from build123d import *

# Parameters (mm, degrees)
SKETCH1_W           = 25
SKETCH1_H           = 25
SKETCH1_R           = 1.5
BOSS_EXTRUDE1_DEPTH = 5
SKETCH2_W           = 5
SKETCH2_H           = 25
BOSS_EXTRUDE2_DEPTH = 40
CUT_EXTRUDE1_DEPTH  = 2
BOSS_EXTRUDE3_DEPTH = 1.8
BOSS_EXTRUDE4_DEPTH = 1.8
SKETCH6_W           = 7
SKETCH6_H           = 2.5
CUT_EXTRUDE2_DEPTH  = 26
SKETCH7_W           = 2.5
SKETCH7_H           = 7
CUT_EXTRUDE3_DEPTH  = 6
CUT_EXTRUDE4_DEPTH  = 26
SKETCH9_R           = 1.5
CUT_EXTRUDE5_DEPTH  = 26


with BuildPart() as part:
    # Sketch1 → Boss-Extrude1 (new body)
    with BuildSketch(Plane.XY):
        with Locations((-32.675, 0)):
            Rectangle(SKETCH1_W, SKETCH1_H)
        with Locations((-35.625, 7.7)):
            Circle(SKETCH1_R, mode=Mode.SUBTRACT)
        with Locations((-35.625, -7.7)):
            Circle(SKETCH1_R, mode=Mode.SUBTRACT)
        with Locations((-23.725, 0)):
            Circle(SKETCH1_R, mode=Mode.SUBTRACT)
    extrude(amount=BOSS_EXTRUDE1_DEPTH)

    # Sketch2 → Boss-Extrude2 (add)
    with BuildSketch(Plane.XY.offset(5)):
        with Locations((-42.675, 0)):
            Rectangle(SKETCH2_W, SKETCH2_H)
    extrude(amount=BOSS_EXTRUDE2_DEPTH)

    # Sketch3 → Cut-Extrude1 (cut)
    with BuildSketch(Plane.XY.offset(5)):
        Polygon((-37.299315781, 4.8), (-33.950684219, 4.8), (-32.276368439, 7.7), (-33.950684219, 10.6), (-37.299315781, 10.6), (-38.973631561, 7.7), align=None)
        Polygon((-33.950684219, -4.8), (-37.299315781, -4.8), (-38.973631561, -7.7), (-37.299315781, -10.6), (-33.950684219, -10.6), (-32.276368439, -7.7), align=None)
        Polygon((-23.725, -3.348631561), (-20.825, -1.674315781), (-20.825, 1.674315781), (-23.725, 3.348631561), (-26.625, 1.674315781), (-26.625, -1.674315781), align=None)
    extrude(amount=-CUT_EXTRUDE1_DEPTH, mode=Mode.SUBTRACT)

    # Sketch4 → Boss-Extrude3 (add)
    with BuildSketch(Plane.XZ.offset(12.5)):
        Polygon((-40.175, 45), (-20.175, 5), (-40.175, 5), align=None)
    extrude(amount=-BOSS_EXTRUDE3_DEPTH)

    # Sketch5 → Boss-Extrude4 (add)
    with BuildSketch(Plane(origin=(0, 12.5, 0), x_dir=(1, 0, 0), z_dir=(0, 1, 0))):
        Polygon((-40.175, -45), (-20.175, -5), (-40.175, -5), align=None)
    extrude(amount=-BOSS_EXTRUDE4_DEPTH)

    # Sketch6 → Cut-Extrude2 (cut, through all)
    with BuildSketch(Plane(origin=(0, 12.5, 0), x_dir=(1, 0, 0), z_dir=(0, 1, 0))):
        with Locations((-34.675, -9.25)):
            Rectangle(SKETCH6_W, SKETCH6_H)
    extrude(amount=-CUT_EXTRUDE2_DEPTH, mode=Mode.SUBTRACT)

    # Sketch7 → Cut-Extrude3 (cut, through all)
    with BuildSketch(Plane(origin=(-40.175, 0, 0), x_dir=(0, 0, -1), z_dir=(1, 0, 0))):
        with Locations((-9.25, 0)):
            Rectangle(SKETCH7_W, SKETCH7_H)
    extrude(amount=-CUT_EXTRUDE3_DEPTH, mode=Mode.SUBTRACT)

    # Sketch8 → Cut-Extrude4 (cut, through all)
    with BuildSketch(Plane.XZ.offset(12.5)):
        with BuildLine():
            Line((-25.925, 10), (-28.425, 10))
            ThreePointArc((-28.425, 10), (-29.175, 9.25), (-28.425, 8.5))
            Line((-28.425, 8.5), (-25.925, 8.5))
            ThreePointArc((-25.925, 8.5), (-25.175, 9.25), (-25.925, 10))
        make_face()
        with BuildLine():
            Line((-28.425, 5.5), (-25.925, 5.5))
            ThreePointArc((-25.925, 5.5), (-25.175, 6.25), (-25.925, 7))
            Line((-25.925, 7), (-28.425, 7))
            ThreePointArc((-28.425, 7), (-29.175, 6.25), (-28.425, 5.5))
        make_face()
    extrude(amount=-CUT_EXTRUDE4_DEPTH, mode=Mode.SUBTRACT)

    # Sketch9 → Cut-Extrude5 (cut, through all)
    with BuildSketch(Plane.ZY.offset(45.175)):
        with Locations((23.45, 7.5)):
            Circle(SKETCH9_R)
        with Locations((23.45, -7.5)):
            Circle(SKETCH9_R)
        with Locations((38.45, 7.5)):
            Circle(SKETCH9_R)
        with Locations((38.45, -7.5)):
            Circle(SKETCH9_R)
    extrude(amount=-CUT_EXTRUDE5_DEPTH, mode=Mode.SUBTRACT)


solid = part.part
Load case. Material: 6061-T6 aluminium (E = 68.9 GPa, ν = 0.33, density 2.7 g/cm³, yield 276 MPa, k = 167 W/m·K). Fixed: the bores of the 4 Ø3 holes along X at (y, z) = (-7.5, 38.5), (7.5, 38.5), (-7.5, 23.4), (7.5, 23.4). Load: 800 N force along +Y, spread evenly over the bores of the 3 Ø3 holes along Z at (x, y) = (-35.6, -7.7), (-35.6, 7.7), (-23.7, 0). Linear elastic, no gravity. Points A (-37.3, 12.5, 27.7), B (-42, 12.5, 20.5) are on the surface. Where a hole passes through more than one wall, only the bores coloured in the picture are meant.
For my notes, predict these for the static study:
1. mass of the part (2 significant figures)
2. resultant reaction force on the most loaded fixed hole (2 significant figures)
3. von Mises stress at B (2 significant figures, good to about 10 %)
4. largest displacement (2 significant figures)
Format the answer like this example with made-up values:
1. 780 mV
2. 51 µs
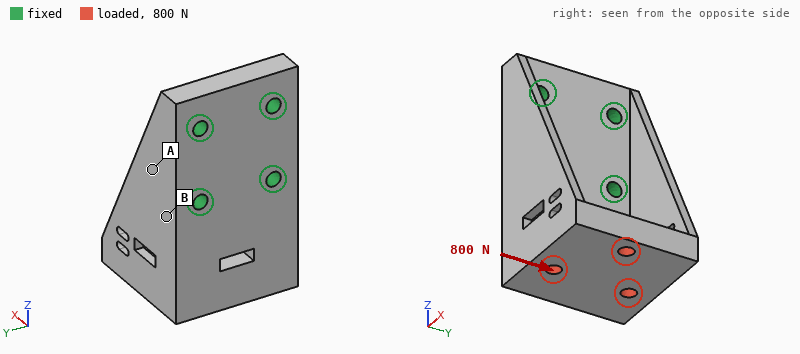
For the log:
1. 24 g
2. 1.2 kN
3. 36 MPa
4. 89 µm
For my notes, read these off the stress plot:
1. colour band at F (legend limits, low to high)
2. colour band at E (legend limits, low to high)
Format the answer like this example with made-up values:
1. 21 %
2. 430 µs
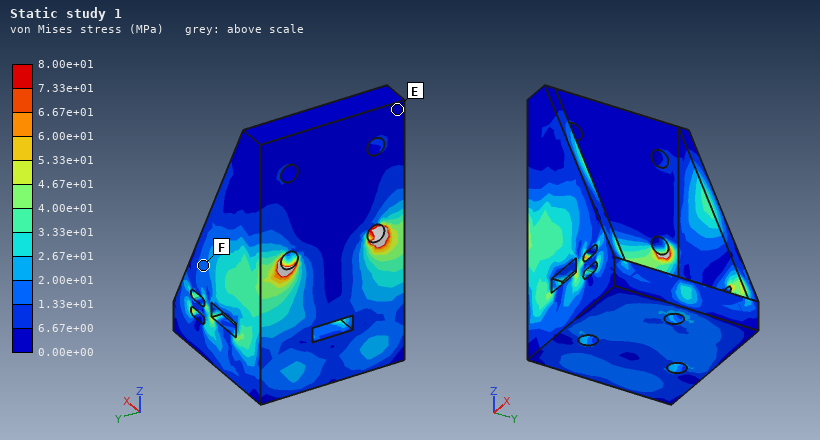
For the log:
1. 1.33e+01 to 2.00e+01 MPa
2. 0.00e+00 to 6.67e+00 MPa
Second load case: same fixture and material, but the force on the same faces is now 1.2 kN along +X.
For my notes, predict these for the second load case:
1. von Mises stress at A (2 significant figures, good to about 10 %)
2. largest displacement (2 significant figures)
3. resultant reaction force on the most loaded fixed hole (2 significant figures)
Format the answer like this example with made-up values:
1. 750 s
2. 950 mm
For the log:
1. 43 MPa
2. 0.11 mm
3. 1.2 kN
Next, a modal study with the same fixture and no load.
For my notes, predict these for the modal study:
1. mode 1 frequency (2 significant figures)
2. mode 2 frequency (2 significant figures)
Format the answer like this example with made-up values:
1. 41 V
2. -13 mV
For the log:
1. 5700 Hz
2. 5900 Hz
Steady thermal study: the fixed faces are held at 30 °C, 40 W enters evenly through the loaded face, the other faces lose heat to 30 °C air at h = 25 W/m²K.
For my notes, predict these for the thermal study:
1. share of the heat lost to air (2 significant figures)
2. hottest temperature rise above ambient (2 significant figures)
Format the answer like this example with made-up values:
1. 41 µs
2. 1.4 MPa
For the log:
1. 7.0 %
2. 52 K
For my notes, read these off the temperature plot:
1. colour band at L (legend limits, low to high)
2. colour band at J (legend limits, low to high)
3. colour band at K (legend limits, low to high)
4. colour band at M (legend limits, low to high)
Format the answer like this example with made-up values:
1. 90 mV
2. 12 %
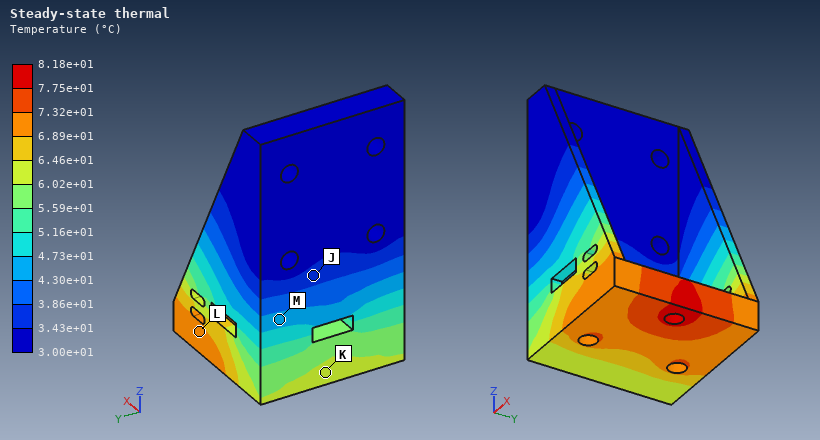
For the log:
1. 6.89e+01 to 7.32e+01 °C
2. 3.43e+01 to 3.86e+01 °C
3. 6.02e+01 to 6.46e+01 °C
4. 4.30e+01 to 4.73e+01 °C
